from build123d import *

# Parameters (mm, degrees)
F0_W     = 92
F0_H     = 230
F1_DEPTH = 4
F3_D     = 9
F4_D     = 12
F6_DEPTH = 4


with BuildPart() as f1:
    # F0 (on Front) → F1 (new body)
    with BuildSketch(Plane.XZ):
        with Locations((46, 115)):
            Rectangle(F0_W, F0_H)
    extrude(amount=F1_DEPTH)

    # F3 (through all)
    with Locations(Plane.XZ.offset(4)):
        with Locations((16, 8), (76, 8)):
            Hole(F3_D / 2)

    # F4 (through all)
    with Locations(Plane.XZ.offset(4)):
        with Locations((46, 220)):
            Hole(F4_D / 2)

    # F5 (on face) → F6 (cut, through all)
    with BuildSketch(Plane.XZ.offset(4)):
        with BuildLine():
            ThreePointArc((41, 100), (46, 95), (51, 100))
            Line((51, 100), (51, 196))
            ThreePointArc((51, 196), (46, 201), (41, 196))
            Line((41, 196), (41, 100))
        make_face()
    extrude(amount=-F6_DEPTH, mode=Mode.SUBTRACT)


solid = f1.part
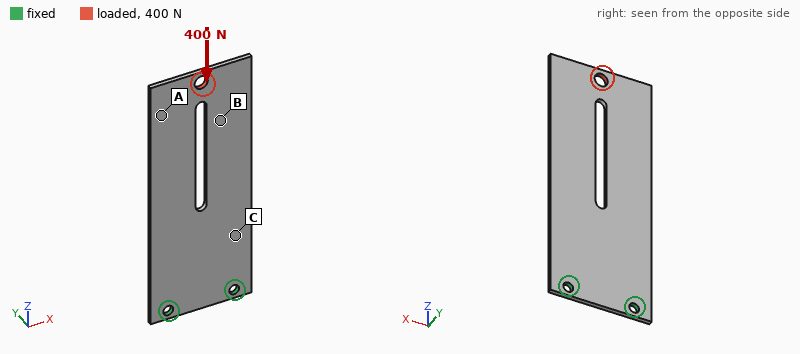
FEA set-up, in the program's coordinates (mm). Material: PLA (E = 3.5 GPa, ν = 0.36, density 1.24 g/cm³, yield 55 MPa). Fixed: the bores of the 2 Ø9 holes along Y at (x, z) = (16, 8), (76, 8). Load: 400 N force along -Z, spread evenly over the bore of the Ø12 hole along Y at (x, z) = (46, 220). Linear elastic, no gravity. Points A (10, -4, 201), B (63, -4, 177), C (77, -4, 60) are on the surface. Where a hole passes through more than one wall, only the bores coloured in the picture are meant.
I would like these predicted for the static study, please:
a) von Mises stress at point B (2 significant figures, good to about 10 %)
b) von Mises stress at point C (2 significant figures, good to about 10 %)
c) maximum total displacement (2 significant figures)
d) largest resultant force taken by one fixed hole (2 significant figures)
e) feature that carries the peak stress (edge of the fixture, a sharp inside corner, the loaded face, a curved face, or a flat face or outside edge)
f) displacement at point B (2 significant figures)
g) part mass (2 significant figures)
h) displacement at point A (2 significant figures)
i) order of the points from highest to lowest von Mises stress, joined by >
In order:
1.8 MPa
1.2 MPa
0.13 mm
200 N
a flat face or outside edge
0.069 mm
99 g
0.062 mm
B > C > A
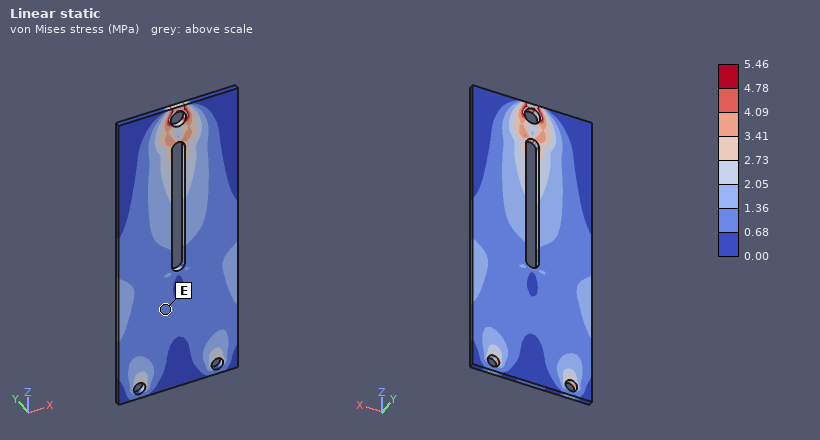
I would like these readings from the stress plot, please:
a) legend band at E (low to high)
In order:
0.68 to 1.36 MPa
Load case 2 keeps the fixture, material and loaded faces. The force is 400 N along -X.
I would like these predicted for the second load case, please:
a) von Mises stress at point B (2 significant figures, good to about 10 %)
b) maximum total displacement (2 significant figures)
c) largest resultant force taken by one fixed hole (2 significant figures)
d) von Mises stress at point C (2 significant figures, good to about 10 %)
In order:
4.7 MPa
2.4 mm
1.3 kN
7.6 MPa
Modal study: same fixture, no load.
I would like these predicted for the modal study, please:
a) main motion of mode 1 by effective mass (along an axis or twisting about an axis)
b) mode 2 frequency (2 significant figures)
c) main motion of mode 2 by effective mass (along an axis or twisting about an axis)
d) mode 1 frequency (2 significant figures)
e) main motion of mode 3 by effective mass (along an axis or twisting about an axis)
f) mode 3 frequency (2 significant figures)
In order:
along Y
110 Hz
twisting about Z
23 Hz
along Y
140 Hz
